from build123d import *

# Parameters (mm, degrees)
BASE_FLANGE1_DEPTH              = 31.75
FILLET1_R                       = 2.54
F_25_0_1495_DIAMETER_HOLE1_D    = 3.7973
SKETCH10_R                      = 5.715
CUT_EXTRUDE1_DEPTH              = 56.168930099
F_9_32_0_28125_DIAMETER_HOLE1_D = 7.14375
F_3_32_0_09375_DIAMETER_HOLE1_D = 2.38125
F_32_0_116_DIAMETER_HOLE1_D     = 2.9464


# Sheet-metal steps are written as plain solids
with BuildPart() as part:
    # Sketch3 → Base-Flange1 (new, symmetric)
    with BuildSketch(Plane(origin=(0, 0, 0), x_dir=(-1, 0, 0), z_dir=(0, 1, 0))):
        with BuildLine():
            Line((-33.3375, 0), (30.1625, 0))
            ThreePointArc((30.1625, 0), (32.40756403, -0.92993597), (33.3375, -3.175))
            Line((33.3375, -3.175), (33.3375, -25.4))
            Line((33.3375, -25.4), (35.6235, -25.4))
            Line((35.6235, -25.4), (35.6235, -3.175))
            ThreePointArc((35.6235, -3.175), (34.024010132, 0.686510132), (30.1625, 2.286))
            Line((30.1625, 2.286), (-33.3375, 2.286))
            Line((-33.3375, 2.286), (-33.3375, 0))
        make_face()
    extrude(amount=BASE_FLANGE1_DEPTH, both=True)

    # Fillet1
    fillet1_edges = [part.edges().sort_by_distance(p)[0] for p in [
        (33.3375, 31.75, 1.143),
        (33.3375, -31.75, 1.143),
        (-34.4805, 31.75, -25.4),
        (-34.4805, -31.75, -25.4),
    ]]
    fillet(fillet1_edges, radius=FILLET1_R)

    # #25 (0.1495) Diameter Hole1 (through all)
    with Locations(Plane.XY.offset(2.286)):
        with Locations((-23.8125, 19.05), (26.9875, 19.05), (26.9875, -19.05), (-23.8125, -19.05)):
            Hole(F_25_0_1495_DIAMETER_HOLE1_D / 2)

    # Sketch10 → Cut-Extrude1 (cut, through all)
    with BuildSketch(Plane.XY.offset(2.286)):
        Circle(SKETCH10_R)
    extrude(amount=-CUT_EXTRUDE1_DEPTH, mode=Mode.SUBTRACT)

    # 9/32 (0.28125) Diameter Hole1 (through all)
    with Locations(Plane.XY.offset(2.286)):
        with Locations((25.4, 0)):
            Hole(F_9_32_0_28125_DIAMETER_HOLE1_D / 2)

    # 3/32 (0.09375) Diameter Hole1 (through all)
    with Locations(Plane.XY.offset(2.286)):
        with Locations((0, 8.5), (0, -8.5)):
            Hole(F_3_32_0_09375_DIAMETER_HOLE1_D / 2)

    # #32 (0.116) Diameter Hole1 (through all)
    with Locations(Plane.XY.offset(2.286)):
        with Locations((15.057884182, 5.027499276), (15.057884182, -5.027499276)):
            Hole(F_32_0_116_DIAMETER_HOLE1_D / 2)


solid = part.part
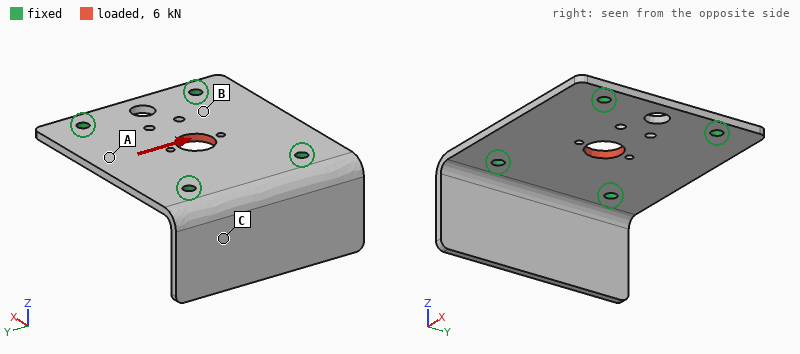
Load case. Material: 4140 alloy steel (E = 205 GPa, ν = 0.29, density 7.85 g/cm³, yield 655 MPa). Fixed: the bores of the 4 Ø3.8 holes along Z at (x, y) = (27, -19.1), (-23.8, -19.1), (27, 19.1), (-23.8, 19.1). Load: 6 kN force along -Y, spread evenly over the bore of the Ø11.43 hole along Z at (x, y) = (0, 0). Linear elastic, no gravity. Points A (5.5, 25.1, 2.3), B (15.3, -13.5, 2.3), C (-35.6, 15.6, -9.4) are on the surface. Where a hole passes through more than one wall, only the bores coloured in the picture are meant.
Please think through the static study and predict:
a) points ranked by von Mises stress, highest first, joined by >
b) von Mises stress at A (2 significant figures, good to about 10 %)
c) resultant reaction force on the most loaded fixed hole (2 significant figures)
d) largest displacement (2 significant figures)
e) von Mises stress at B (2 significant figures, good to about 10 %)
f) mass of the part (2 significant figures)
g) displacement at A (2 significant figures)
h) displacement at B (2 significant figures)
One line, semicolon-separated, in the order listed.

B > A > C; 23 MPa; 1.8 kN; 11 µm; 46 MPa; 100 g; 6.8 µm; 4.8 µm
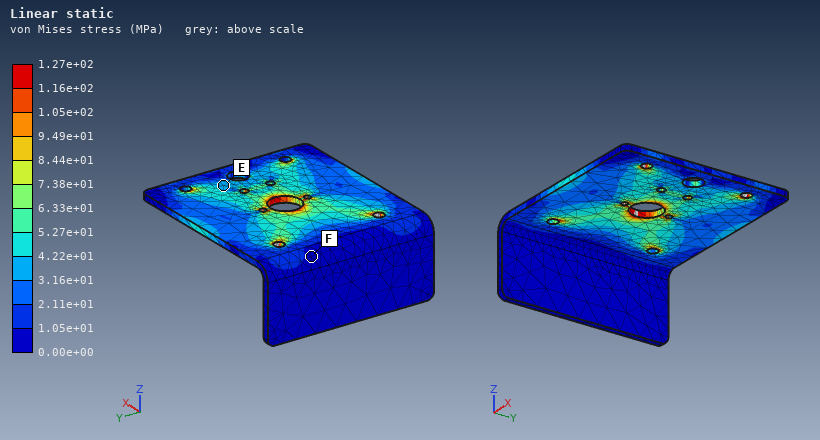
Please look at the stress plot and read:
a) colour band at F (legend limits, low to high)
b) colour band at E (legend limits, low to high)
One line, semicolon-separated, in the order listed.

0.00e+00 to 1.05e+01 MPa; 3.16e+01 to 4.22e+01 MPa
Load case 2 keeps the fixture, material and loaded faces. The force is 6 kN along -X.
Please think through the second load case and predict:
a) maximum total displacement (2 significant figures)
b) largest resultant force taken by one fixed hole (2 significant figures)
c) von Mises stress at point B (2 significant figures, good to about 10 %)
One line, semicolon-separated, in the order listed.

8.4 µm; 1.7 kN; 43 MPa
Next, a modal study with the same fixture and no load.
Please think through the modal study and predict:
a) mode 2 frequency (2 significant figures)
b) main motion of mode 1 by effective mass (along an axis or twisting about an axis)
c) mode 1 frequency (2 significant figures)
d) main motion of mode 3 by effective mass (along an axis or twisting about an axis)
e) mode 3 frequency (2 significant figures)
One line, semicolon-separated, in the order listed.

2800 Hz; along X; 1700 Hz; along Z; 4100 Hz
